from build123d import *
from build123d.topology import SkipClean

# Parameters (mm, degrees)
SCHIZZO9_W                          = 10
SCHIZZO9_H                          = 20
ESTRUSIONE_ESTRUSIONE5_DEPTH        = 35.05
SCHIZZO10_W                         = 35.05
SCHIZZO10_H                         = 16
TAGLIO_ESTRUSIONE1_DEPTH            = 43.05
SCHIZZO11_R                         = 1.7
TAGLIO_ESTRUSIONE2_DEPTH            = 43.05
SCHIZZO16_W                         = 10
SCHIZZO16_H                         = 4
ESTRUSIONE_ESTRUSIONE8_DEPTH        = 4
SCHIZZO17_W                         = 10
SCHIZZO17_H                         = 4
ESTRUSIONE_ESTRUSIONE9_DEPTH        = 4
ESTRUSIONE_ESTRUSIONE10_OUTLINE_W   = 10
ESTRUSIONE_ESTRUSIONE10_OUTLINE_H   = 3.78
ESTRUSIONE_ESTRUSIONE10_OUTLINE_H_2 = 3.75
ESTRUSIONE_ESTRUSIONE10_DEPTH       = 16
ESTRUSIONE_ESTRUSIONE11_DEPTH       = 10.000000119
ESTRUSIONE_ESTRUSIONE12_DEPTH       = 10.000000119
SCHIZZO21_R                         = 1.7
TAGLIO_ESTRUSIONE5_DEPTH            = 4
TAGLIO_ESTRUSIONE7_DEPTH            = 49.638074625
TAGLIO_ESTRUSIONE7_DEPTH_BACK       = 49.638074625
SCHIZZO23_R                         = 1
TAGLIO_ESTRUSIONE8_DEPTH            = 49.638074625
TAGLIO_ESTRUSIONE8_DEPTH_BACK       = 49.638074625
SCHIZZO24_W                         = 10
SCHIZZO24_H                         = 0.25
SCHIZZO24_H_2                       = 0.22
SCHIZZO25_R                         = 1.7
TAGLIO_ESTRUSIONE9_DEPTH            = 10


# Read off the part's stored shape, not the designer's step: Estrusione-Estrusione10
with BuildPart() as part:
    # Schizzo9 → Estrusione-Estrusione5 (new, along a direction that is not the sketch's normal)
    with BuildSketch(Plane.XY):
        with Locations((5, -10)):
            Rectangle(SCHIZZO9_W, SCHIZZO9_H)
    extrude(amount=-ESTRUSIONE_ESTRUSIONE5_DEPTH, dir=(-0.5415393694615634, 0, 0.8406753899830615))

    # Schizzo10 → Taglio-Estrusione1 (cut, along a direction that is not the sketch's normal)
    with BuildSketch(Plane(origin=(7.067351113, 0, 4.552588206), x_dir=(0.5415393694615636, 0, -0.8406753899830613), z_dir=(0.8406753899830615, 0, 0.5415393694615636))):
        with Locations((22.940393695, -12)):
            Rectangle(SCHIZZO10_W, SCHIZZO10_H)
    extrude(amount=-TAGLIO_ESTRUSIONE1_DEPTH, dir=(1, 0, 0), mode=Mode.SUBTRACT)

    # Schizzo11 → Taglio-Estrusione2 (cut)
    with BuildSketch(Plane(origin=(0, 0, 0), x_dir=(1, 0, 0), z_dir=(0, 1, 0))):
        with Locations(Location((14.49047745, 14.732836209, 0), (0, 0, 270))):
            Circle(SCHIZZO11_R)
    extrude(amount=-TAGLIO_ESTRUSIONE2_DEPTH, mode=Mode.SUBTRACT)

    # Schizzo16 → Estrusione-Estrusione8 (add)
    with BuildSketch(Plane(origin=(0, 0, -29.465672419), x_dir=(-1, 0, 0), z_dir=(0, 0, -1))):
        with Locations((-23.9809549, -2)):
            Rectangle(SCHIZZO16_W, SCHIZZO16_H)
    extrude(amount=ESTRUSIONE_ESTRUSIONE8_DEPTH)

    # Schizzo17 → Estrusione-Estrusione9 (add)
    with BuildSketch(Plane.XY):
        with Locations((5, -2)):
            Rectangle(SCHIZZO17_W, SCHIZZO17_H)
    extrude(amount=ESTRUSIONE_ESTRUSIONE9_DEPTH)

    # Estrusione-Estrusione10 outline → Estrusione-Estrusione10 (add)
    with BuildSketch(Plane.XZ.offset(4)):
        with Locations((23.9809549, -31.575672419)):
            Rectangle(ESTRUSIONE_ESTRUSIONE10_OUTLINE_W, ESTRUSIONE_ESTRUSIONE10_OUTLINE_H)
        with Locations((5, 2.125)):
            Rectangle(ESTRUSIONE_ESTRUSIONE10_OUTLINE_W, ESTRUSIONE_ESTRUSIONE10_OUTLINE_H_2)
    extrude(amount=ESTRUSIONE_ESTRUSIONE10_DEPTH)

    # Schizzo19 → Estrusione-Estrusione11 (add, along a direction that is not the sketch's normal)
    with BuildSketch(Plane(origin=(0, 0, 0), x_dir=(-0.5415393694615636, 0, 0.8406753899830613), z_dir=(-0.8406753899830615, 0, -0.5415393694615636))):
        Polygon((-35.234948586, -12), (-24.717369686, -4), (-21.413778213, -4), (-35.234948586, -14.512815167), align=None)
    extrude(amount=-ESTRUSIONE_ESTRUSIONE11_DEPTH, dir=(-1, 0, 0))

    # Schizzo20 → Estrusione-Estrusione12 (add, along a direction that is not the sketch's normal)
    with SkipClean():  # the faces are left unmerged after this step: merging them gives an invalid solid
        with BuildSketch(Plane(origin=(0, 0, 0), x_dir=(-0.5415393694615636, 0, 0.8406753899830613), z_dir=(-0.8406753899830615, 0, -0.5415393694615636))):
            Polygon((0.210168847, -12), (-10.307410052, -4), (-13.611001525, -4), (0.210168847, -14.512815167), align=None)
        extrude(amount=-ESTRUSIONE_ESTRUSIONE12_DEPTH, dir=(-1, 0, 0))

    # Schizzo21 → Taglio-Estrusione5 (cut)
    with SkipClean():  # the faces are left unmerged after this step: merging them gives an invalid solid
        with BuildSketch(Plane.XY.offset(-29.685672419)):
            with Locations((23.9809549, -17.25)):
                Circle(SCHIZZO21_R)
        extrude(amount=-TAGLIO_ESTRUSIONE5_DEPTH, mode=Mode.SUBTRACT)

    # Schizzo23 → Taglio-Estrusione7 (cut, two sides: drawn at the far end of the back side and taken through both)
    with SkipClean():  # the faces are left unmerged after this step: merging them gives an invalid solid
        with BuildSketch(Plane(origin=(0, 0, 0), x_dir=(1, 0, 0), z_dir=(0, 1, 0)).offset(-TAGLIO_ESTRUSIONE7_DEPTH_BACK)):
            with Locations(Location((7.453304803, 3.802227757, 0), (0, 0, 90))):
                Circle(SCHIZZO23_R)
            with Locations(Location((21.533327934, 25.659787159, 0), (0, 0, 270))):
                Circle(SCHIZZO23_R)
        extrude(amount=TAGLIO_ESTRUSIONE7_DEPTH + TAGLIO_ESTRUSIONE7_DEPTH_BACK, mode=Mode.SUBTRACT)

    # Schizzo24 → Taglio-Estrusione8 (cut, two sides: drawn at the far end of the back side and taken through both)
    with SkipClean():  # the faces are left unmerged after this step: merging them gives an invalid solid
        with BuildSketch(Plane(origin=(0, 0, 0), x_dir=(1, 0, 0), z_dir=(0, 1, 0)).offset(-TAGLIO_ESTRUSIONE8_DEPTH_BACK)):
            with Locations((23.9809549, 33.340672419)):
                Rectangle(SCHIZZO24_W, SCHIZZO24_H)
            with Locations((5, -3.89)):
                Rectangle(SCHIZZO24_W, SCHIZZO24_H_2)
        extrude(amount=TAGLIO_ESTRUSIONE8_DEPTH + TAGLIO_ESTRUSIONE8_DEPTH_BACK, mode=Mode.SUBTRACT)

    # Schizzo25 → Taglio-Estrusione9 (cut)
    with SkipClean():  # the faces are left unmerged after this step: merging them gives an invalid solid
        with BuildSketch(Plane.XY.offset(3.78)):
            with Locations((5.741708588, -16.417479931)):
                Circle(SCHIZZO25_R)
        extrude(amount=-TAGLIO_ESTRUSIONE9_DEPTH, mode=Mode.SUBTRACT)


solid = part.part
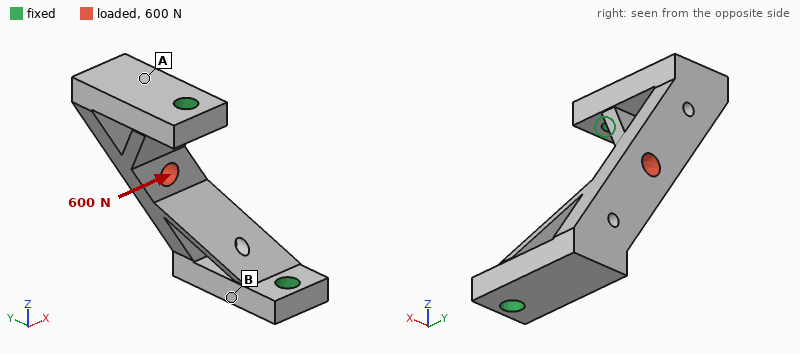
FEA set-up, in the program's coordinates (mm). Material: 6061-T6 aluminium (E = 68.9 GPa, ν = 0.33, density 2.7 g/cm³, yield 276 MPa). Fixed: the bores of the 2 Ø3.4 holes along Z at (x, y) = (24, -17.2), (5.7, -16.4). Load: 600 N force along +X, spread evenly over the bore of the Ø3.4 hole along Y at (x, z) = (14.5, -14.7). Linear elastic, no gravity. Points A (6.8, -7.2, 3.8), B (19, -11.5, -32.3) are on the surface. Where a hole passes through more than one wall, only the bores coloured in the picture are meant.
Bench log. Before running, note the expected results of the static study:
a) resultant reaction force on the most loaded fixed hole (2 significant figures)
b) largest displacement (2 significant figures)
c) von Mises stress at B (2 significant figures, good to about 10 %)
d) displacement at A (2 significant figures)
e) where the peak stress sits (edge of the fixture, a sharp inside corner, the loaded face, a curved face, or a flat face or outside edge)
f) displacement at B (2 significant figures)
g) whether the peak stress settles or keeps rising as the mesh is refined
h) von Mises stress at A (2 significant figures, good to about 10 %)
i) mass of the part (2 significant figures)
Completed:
300 N
82 µm
55 MPa
16 µm
edge of the fixture
16 µm
keeps rising
19 MPa
8.1 g
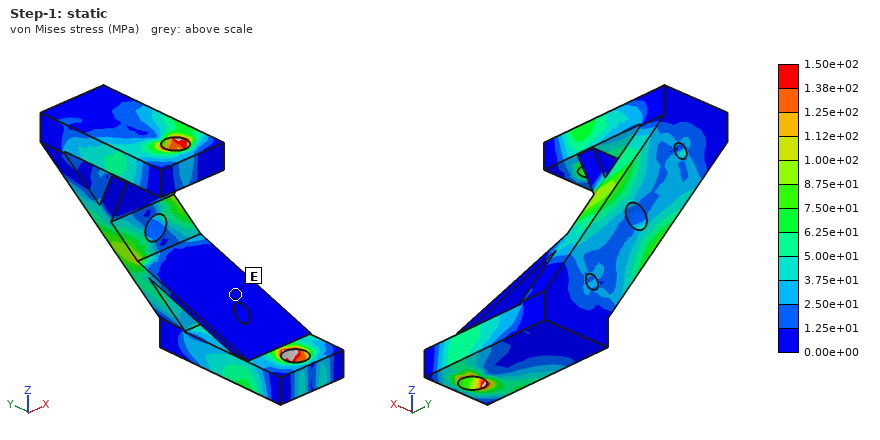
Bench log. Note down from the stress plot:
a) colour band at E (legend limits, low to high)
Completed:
0.00e+00 to 1.25e+01 MPa
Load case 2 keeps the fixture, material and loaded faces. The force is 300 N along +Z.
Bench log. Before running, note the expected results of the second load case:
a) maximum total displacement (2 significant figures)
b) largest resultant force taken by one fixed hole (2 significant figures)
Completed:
38 µm
160 N
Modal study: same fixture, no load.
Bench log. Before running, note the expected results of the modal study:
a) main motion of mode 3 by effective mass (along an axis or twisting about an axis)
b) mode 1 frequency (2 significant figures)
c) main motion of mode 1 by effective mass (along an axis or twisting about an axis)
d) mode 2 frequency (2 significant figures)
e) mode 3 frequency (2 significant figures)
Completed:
along X
5700 Hz
along Z
6700 Hz
7600 Hz
